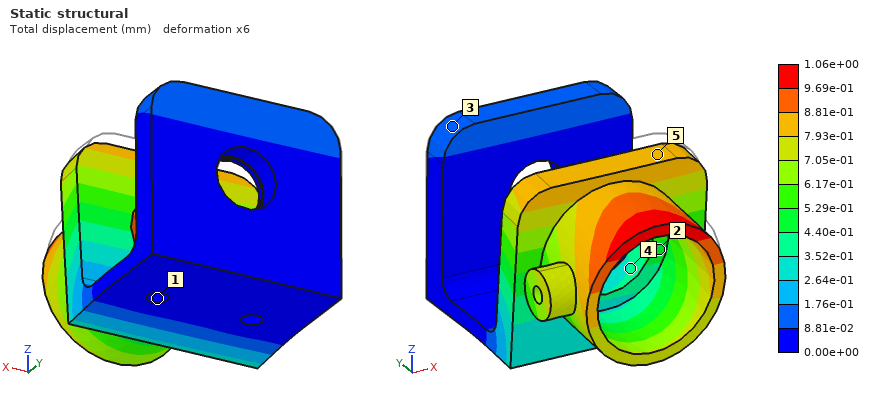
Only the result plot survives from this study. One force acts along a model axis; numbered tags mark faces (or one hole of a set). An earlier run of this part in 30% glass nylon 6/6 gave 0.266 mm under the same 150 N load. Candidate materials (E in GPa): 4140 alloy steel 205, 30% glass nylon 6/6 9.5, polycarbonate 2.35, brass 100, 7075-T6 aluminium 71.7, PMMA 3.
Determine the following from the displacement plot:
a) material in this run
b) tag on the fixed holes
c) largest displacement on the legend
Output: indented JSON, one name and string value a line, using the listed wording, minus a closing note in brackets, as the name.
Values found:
{
  "material in this run": "polycarbonate",
  "tag on the fixed holes": "1",
  "largest displacement on the legend": "1.06e+00 mm"
}
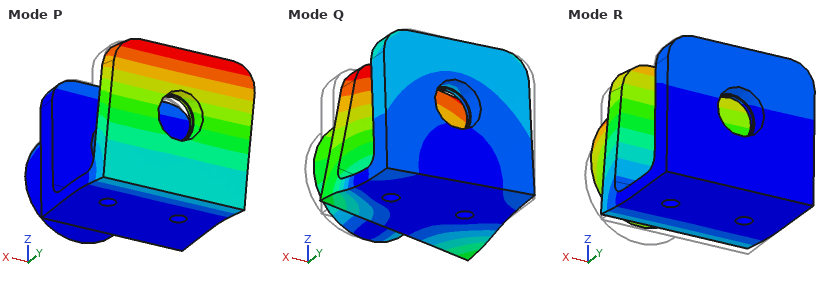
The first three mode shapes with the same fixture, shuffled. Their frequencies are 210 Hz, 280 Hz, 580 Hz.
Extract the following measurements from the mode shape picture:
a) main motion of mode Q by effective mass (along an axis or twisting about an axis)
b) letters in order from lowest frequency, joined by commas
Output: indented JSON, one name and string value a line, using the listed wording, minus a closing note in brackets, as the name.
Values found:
{
  "main motion of mode Q by effective mass": "along X",
  "letters in order from lowest frequency, joined by commas": "R, P, Q"
}
